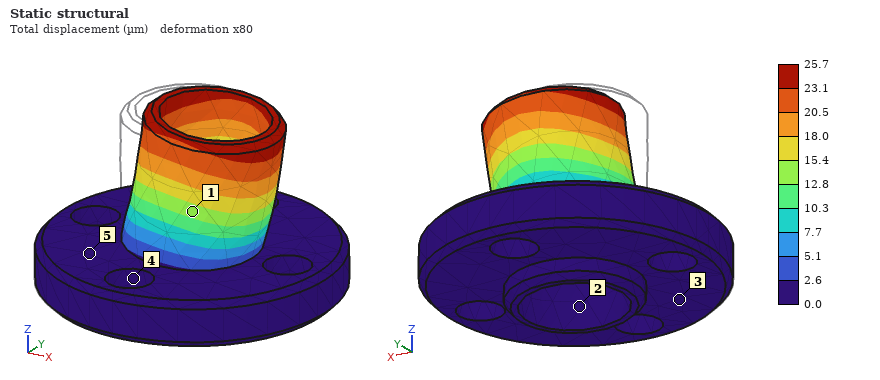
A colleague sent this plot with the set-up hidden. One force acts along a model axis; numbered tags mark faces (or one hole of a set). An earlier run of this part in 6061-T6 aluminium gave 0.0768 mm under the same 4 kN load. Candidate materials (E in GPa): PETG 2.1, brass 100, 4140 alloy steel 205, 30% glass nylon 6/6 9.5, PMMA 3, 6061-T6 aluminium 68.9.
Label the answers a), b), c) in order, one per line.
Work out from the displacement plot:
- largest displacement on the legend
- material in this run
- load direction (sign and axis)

a) 25.7 µm
b) 4140 alloy steel
c) +X
